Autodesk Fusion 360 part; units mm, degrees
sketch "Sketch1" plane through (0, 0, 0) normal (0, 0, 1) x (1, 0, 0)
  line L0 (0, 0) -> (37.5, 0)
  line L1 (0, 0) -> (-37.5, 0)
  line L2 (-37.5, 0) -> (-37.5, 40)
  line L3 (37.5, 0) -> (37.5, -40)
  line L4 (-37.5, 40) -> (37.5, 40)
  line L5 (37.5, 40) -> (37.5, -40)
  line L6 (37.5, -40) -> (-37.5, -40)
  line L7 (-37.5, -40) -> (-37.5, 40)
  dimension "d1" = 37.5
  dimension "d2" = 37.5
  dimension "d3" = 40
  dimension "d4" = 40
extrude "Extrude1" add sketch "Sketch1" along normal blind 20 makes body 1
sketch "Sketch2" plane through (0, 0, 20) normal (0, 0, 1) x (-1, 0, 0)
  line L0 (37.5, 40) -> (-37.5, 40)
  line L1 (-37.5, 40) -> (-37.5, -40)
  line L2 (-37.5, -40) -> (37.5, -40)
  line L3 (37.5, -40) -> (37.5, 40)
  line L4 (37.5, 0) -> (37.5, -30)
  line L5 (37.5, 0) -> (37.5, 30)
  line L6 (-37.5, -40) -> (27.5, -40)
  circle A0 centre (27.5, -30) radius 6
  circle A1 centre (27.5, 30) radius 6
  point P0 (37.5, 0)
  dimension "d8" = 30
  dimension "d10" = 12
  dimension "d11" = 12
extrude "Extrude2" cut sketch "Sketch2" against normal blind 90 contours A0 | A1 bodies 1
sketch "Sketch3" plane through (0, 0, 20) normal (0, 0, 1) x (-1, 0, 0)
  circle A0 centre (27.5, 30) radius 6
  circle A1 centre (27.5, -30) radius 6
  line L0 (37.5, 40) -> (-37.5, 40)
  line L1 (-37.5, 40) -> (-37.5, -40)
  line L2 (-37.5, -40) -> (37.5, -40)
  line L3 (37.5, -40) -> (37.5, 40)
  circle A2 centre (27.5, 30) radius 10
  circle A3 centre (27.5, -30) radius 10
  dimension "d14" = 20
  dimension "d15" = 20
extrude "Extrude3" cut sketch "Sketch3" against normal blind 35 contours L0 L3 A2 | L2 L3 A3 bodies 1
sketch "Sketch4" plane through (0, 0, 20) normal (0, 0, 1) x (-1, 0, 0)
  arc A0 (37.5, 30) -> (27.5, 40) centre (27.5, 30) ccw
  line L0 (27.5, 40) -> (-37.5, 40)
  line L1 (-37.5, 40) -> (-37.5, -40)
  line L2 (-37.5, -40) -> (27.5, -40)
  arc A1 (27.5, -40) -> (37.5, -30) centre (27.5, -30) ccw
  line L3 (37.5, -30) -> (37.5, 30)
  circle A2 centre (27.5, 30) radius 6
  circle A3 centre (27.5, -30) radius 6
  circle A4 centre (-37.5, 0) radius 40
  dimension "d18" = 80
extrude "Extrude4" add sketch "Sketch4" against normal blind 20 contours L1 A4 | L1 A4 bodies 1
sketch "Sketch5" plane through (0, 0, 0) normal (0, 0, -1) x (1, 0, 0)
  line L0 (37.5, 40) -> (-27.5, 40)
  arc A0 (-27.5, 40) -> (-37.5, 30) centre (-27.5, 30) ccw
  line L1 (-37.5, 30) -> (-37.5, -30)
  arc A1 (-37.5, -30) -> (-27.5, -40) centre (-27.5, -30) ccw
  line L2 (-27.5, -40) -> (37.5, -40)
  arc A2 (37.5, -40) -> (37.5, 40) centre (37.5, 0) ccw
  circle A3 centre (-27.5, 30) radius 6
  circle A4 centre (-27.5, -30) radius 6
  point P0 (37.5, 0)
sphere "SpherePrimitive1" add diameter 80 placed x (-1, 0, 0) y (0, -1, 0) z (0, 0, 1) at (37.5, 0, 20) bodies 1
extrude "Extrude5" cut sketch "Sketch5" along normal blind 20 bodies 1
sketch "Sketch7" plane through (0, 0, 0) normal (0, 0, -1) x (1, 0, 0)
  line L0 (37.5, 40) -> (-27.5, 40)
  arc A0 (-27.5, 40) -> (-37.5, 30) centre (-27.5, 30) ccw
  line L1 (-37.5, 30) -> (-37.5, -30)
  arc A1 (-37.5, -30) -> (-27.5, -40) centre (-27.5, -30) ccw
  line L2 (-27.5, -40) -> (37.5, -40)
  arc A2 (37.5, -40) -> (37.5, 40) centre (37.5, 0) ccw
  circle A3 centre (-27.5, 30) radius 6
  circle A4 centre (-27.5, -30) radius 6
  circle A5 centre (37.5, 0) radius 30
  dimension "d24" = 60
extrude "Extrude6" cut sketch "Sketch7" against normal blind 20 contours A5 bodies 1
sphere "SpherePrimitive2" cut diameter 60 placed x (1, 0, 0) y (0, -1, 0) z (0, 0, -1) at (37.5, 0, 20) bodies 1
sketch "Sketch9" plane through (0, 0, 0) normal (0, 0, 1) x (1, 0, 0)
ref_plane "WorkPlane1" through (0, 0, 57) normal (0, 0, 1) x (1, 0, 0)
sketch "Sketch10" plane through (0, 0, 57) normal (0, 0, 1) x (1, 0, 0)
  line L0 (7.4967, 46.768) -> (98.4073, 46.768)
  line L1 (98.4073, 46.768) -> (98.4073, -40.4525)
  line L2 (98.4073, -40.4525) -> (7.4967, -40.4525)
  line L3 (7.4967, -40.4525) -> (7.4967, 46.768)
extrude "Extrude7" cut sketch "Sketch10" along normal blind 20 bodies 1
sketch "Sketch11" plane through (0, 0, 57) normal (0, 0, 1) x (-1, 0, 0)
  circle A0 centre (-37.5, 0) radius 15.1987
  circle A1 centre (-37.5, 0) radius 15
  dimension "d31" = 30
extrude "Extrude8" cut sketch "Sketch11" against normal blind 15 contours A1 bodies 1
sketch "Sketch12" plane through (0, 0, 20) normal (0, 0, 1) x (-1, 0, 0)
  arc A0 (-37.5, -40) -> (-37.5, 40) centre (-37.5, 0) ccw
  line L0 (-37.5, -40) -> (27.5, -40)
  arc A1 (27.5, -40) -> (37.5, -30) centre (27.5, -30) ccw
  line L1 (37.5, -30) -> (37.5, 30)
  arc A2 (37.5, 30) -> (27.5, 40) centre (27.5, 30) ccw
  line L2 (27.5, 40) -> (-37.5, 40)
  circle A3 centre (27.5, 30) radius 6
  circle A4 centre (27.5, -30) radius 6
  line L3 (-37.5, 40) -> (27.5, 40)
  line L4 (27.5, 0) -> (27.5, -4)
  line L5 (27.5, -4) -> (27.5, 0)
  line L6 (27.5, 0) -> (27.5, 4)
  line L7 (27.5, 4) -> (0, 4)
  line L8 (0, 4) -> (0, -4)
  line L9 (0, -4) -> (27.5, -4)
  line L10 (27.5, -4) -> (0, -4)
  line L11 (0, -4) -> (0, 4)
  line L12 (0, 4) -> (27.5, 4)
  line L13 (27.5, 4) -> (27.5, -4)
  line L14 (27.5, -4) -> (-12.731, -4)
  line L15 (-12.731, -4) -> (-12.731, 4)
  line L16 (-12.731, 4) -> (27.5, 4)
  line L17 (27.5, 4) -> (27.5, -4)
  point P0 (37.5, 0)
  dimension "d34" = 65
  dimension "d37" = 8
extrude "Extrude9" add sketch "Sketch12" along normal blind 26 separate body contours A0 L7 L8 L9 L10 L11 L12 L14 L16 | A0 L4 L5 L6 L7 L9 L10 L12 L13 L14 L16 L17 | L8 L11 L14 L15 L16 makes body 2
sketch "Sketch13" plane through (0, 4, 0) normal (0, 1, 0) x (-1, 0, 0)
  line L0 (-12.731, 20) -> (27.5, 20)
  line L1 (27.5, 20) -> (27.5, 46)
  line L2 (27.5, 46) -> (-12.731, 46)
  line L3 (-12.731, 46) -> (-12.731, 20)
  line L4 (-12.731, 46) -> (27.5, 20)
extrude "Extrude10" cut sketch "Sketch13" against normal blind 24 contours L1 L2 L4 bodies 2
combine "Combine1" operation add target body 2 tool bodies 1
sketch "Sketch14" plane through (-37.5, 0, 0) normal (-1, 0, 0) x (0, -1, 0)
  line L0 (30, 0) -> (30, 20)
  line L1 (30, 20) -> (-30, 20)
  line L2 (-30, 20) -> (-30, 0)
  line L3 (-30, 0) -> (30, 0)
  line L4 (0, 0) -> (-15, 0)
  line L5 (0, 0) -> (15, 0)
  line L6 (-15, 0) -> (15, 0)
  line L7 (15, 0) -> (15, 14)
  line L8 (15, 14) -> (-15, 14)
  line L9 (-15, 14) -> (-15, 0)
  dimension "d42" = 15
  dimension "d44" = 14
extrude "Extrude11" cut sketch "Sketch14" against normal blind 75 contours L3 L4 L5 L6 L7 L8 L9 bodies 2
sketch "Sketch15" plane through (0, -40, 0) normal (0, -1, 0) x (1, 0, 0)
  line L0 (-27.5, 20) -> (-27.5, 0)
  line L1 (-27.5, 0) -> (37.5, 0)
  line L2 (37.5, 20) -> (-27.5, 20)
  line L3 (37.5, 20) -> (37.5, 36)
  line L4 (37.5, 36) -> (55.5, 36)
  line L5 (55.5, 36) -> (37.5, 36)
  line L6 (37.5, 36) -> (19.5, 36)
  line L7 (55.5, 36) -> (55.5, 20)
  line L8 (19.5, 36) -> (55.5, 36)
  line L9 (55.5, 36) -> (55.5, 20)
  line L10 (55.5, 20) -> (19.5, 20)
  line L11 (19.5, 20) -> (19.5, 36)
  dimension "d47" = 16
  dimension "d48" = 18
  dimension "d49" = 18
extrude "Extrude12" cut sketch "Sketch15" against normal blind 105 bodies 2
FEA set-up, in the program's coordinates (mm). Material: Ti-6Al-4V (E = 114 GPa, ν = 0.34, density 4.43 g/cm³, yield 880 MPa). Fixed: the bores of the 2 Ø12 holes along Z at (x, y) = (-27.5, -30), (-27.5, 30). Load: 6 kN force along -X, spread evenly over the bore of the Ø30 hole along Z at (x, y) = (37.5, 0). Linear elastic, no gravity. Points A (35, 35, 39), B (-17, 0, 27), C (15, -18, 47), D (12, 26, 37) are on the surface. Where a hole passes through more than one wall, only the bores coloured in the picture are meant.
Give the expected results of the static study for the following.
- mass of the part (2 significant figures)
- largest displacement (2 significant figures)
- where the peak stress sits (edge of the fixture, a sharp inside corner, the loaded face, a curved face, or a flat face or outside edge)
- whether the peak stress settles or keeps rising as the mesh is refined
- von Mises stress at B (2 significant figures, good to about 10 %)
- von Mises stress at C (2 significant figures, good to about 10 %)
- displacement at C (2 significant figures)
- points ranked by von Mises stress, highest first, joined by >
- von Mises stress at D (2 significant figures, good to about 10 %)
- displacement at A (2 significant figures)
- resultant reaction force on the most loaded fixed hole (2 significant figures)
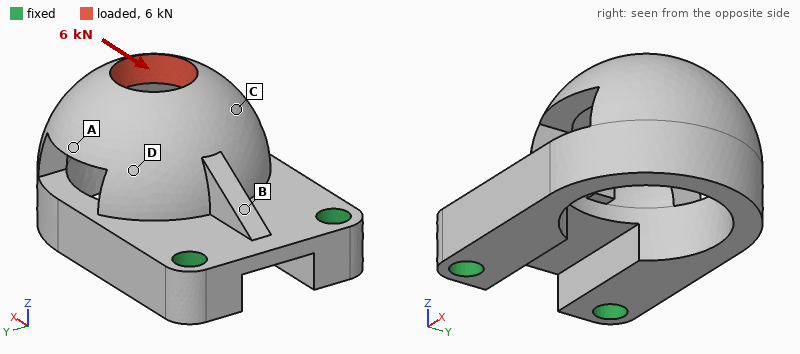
660 g
0.19 mm
edge of the fixture
keeps rising
78 MPa
16 MPa
0.094 mm
B > D > C > A
25 MPa
0.11 mm
3.9 kN
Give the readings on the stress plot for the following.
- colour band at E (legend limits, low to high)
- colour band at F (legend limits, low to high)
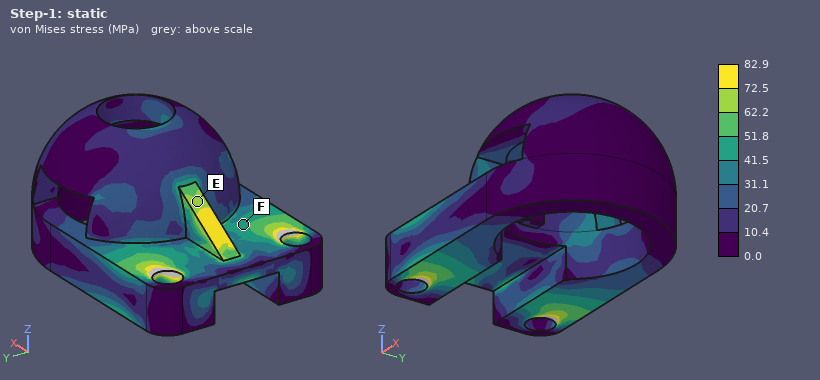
62.2 to 72.5 MPa
41.5 to 51.8 MPa
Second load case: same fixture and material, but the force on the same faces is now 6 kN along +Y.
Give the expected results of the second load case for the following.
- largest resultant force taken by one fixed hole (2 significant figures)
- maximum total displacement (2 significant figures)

7.7 kN
70 µm
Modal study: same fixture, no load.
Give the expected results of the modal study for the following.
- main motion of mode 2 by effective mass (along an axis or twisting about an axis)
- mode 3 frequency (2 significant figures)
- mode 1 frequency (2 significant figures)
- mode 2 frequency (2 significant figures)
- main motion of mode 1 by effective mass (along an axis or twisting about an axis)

along Y
3600 Hz
1400 Hz
2500 Hz
along Z
